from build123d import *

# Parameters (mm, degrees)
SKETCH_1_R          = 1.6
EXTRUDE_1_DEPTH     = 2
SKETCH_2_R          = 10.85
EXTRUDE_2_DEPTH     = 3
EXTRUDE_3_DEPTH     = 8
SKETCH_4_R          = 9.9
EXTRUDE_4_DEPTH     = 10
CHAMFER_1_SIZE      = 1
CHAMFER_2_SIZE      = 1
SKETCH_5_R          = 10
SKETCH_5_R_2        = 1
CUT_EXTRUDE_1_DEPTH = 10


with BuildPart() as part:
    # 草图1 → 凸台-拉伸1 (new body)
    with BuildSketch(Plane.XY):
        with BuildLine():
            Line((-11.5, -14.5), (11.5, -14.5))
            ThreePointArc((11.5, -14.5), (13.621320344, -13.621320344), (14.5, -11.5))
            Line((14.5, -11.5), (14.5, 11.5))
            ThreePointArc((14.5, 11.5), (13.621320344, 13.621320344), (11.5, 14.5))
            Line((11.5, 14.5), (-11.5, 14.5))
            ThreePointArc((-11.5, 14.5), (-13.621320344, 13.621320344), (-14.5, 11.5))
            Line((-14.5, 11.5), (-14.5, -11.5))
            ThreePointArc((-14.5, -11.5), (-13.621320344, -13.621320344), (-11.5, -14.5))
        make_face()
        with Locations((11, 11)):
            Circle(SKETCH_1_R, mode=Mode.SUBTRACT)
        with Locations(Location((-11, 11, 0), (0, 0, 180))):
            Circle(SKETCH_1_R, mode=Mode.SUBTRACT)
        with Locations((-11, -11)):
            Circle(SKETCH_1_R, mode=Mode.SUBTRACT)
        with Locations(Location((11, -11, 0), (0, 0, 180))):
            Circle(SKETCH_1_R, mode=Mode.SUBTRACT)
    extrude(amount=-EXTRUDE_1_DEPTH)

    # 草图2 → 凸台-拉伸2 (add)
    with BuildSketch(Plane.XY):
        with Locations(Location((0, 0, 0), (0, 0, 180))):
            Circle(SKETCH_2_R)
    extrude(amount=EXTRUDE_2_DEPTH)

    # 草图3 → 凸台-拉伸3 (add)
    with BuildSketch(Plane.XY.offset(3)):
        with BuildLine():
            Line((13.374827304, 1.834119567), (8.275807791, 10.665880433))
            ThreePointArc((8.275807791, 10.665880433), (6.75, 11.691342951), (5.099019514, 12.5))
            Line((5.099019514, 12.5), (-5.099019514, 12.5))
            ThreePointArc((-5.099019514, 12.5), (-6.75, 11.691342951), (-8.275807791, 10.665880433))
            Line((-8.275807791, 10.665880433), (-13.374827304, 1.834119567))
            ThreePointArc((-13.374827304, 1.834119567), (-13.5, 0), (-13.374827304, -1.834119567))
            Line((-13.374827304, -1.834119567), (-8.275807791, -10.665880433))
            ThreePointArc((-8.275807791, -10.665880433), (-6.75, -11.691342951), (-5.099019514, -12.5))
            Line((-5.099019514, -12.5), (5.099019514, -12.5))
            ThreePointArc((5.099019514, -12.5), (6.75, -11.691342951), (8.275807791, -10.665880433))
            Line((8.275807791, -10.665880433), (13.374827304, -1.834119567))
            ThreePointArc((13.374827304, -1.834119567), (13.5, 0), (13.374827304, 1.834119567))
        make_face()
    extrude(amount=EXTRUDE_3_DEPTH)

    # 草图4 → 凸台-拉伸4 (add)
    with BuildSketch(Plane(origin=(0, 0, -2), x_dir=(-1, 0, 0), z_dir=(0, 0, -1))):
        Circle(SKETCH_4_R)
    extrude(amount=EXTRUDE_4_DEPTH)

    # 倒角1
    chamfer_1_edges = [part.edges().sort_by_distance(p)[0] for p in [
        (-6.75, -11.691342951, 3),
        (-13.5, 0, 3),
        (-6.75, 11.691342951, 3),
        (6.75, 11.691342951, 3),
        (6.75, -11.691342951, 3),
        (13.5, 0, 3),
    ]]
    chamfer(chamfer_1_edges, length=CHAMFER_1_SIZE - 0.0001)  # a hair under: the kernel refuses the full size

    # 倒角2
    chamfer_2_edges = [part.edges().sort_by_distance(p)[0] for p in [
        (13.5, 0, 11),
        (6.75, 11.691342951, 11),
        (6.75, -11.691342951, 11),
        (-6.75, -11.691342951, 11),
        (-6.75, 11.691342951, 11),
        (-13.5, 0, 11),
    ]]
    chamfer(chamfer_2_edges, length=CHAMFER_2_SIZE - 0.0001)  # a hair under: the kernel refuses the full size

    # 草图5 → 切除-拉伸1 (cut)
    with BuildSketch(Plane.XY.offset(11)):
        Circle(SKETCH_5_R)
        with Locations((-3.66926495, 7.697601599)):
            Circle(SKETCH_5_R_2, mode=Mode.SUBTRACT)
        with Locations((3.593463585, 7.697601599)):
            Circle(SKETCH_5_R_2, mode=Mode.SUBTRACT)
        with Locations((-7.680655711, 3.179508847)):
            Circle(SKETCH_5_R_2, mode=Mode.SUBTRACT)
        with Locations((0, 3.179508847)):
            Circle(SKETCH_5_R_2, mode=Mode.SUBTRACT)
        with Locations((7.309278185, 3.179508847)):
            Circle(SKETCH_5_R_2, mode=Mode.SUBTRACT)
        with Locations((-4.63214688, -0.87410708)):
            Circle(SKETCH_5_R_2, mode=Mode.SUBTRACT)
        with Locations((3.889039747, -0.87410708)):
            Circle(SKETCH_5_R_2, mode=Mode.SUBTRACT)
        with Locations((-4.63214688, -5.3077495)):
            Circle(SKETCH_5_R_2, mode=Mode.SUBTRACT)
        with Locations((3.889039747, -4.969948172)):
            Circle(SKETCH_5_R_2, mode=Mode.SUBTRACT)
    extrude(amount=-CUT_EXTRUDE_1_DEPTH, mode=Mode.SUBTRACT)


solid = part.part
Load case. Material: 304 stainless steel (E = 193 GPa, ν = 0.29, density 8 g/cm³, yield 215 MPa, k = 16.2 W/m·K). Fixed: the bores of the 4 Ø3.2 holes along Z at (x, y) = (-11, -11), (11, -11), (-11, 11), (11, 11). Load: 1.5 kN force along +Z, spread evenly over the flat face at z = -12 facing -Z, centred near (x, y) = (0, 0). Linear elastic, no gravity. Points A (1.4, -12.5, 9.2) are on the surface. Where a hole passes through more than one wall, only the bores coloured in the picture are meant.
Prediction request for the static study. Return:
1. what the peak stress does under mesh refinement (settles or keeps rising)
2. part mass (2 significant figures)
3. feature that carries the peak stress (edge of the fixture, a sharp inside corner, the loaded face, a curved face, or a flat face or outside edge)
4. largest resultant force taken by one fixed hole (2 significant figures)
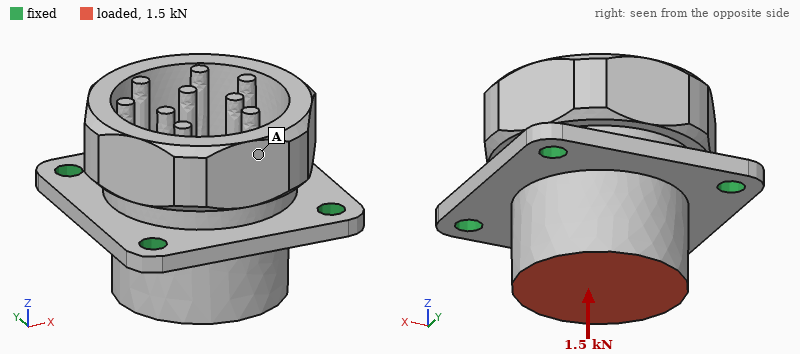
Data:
keeps rising
57 g
edge of the fixture
380 N
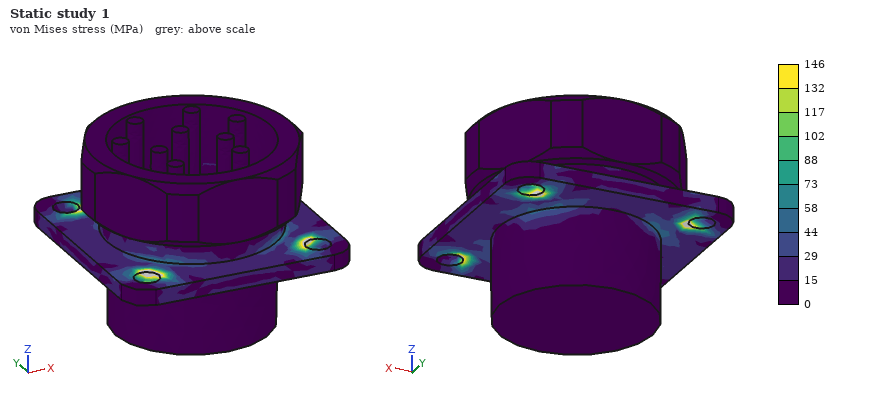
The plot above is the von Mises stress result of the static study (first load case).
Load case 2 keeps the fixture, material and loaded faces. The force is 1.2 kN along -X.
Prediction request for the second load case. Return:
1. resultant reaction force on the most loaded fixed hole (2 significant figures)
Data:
470 N
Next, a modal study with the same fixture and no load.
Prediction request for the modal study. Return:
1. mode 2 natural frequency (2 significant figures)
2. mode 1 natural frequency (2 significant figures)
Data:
11 kHz
11 kHz
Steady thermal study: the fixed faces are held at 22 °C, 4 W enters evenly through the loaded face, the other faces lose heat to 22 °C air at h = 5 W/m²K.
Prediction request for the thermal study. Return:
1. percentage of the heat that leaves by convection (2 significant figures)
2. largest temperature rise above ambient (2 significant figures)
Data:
7.4 %
25 K
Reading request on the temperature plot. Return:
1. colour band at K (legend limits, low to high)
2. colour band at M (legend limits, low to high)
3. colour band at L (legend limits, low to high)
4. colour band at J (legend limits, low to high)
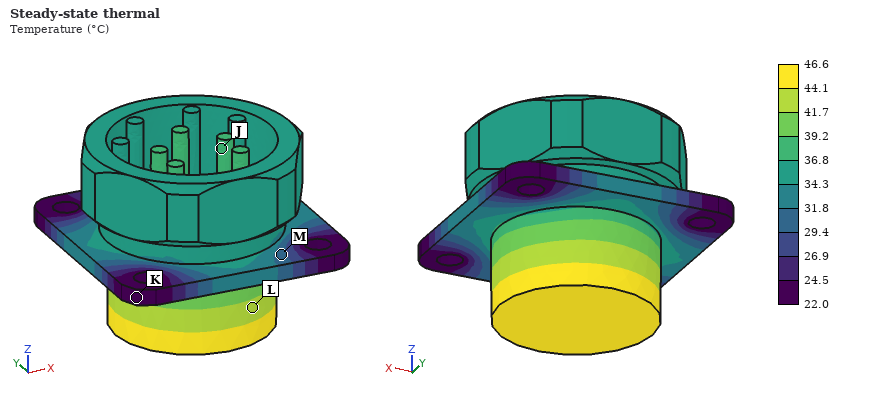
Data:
22.0 to 24.5 °C
29.4 to 31.8 °C
41.7 to 44.1 °C
36.8 to 39.2 °C
